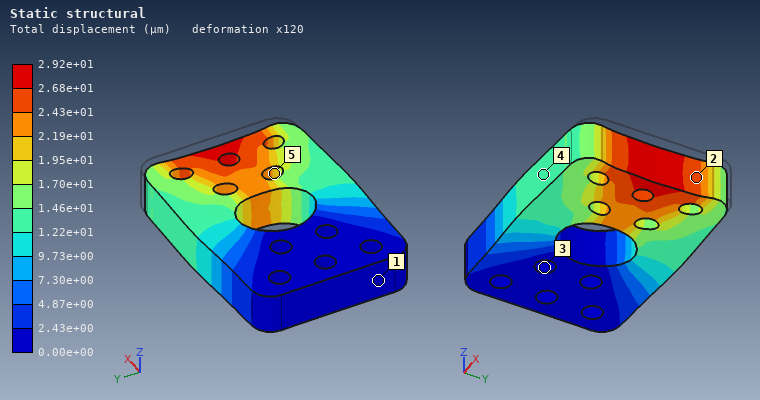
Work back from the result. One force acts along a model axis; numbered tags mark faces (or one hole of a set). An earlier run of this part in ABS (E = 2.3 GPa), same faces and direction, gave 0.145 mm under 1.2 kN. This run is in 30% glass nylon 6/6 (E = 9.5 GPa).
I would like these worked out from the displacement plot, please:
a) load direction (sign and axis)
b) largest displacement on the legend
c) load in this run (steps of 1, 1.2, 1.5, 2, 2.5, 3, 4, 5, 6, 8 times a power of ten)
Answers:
-X
2.92e+01 µm
1 kN
